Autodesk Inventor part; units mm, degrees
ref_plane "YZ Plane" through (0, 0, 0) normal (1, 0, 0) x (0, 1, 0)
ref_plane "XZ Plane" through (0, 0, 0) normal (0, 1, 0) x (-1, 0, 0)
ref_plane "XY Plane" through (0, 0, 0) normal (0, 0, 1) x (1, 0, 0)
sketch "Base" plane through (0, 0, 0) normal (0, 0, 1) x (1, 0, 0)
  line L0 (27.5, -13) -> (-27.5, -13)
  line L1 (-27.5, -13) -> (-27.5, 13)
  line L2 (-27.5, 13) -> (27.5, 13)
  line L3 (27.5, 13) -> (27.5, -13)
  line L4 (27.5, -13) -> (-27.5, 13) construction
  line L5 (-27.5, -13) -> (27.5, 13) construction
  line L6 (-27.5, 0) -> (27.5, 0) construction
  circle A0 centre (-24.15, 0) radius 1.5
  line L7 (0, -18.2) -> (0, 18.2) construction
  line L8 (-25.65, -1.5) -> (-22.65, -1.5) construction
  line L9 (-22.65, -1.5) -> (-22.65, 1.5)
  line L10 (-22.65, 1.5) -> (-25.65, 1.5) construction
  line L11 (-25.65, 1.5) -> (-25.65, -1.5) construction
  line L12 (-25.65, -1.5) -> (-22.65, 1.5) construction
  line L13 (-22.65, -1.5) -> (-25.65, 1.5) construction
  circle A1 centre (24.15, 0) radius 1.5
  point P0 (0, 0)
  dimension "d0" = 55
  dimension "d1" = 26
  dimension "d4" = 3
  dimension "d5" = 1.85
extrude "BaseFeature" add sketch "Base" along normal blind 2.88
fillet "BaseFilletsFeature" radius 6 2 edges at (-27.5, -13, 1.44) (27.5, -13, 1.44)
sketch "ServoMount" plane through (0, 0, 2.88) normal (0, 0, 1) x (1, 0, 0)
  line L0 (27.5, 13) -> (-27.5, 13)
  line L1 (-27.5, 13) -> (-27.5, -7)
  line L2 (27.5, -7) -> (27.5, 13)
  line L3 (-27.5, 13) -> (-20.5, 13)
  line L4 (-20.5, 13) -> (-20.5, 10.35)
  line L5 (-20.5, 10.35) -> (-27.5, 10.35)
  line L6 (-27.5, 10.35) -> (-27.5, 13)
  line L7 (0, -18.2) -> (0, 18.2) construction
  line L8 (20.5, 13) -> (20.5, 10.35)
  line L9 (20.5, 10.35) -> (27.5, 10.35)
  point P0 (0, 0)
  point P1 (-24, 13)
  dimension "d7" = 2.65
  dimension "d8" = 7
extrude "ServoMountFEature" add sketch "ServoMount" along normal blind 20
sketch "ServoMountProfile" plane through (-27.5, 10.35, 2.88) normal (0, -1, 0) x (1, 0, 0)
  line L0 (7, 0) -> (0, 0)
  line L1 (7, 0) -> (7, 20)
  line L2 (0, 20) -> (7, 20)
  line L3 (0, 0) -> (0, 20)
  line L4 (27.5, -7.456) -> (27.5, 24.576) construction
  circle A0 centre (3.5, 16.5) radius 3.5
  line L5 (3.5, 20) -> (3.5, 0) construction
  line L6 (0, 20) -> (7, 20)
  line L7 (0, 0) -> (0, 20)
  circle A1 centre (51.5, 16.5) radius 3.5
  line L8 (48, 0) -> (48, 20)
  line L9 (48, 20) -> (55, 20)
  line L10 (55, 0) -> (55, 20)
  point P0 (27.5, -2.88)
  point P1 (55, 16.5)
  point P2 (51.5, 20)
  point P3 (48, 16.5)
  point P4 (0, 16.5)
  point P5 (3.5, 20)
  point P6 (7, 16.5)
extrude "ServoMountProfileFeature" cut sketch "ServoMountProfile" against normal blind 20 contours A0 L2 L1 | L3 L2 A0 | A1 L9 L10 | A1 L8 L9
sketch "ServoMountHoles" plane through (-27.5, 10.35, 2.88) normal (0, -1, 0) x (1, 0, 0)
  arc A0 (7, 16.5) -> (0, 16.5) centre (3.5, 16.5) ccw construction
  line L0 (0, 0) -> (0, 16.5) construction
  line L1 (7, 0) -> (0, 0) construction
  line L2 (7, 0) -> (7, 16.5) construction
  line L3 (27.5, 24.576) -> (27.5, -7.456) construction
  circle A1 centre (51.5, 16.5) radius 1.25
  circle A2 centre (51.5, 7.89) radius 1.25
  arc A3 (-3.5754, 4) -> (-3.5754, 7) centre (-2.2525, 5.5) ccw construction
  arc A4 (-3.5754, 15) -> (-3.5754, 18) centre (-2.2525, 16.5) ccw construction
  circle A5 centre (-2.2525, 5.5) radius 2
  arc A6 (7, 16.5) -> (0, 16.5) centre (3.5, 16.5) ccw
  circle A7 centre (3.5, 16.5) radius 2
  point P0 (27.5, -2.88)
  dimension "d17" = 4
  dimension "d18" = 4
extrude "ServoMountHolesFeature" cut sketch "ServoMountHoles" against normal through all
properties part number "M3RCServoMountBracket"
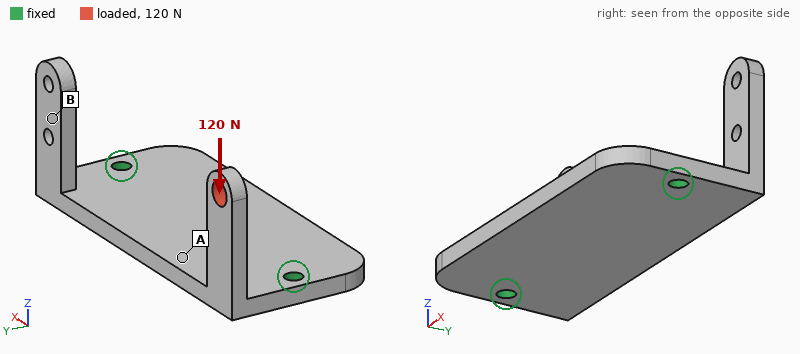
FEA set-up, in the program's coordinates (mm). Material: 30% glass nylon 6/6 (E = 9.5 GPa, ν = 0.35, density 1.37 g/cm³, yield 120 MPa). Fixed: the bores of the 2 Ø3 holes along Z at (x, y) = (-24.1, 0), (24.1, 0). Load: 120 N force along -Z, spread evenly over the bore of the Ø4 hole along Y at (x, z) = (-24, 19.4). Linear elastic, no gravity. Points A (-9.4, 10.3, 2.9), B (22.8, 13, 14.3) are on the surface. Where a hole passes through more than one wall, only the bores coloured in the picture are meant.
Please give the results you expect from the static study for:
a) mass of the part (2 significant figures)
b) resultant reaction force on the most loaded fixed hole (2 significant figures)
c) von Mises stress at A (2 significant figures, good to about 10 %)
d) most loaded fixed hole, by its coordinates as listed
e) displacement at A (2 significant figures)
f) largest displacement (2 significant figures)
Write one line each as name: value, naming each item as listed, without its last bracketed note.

mass of the part: 6.4 g
resultant reaction force on the most loaded fixed hole: 120 N
von Mises stress at A: 12 MPa
most loaded fixed hole, by its coordinates as listed: (-24.1, 0)
displacement at A: 0.12 mm
largest displacement: 0.69 mm
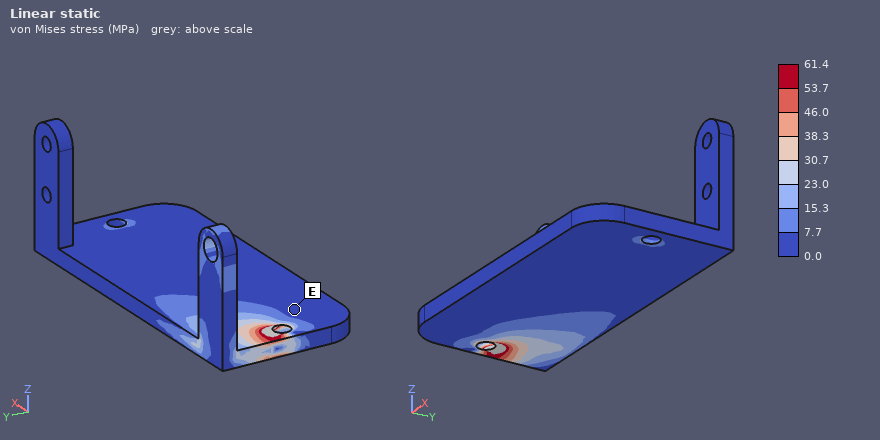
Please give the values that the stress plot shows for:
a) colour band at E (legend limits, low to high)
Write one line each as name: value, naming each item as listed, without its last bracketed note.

colour band at E: 0.0 to 7.7 MPa
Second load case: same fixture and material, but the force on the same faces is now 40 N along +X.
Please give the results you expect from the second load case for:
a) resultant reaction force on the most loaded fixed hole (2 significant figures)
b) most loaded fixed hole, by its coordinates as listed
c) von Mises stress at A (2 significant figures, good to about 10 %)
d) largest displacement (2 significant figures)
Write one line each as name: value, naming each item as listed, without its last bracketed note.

resultant reaction force on the most loaded fixed hole: 29 N
most loaded fixed hole, by its coordinates as listed: (-24.1, 0)
von Mises stress at A: 8.8 MPa
largest displacement: 0.62 mm
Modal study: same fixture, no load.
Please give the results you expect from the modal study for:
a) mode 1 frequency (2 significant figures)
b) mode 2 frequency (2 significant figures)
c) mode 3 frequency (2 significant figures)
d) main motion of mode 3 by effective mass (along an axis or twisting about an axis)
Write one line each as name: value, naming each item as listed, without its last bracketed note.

mode 1 frequency: 1900 Hz
mode 2 frequency: 2100 Hz
mode 3 frequency: 2500 Hz
main motion of mode 3 by effective mass: along Z
